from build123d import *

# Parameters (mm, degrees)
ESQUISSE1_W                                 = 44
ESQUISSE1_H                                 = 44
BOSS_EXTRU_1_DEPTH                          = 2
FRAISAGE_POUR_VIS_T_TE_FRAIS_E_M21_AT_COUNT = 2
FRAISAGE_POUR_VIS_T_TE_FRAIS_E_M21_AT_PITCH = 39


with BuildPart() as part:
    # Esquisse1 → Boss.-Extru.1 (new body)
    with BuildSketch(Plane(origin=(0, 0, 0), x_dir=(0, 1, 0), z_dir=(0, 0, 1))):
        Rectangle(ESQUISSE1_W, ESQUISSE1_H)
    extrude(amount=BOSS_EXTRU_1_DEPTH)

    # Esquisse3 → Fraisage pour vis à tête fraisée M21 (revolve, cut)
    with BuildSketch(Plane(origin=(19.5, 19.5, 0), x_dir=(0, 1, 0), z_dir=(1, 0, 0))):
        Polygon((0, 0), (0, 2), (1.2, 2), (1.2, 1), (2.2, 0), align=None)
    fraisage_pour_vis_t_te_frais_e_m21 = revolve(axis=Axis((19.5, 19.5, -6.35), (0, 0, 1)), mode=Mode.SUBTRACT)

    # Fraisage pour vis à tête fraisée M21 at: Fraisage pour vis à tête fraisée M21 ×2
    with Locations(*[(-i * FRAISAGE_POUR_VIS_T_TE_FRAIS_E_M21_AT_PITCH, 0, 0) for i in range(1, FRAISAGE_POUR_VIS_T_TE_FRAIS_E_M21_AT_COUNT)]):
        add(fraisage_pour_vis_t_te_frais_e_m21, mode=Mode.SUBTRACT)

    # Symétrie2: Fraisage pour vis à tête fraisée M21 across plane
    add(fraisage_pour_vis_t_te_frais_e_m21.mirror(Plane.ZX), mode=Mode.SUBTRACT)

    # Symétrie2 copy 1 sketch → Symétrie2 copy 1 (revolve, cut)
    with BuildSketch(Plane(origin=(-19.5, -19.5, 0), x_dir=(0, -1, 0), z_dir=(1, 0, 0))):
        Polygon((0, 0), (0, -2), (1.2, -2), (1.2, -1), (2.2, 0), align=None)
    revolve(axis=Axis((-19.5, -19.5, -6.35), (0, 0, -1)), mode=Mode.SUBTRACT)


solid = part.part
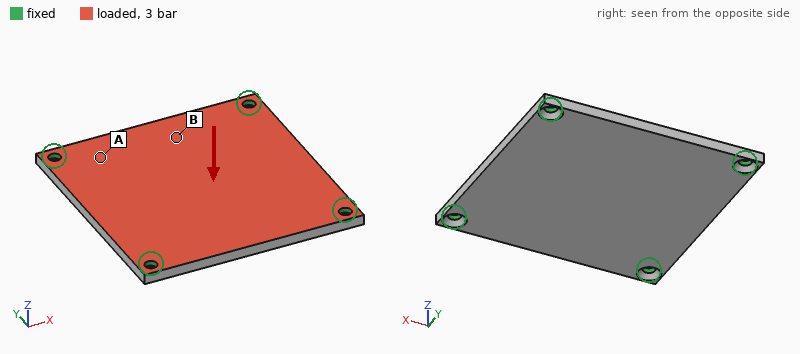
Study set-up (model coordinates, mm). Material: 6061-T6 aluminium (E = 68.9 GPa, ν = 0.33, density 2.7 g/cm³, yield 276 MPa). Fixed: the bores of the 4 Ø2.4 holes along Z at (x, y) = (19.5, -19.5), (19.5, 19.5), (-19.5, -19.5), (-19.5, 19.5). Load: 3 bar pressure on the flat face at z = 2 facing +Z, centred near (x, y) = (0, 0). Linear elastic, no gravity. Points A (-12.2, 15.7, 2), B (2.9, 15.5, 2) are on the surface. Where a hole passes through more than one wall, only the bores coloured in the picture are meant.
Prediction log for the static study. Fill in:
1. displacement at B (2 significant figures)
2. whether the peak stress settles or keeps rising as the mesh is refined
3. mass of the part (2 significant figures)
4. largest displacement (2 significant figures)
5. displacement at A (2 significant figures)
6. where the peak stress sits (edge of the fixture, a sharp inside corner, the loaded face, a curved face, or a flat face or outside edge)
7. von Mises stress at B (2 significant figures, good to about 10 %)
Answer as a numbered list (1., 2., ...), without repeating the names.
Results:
1. 0.092 mm
2. keeps rising
3. 10 g
4. 0.14 mm
5. 0.053 mm
6. edge of the fixture
7. 37 MPa
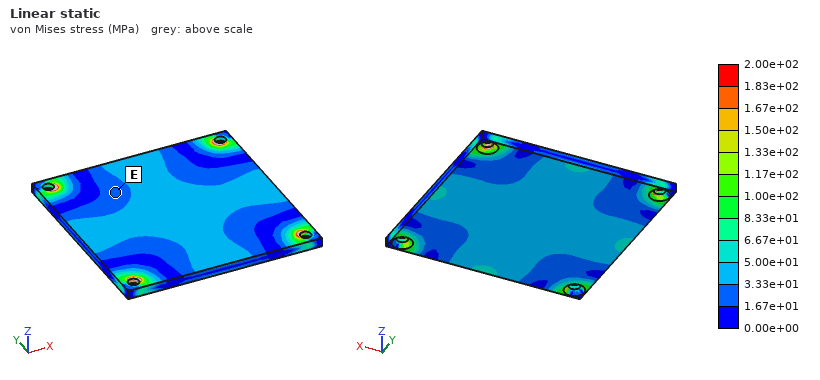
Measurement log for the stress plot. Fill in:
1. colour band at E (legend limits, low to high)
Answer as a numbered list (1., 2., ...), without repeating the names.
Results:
1. 1.67e+01 to 3.33e+01 MPa
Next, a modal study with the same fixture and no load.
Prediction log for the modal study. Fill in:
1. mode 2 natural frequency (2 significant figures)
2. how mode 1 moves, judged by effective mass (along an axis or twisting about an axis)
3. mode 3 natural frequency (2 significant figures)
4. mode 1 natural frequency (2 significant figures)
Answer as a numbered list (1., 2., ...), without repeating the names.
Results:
1. 6800 Hz
2. along Z
3. 6800 Hz
4. 3900 Hz
